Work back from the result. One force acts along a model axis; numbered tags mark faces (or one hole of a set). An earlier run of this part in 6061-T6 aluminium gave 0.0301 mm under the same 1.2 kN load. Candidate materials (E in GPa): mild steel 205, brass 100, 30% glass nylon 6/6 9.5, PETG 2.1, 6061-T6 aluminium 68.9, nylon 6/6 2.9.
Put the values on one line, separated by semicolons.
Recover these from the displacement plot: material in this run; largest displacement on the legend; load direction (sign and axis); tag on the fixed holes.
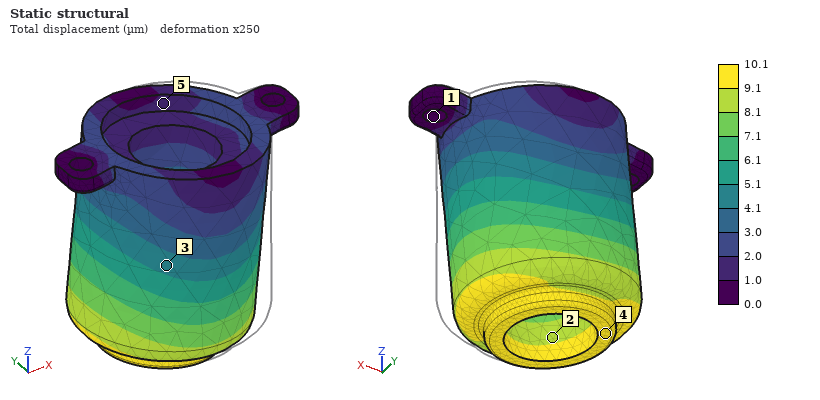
mild steel; 10.1 µm; -X; 1
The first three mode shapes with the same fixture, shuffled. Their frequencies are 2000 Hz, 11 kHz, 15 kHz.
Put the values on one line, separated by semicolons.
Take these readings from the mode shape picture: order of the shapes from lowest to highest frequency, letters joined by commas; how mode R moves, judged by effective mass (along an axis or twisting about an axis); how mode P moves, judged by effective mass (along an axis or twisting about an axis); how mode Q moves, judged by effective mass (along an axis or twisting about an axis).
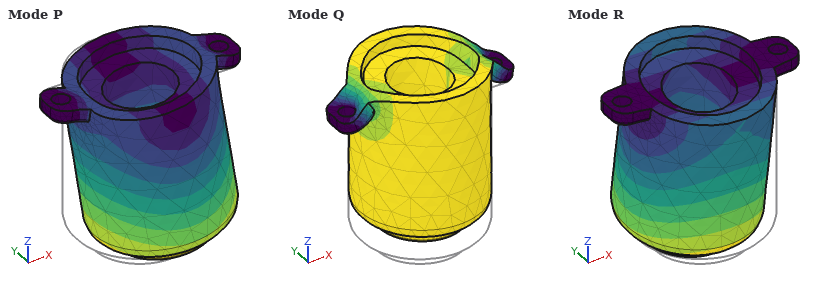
R, P, Q; along Y; along X; along Z
